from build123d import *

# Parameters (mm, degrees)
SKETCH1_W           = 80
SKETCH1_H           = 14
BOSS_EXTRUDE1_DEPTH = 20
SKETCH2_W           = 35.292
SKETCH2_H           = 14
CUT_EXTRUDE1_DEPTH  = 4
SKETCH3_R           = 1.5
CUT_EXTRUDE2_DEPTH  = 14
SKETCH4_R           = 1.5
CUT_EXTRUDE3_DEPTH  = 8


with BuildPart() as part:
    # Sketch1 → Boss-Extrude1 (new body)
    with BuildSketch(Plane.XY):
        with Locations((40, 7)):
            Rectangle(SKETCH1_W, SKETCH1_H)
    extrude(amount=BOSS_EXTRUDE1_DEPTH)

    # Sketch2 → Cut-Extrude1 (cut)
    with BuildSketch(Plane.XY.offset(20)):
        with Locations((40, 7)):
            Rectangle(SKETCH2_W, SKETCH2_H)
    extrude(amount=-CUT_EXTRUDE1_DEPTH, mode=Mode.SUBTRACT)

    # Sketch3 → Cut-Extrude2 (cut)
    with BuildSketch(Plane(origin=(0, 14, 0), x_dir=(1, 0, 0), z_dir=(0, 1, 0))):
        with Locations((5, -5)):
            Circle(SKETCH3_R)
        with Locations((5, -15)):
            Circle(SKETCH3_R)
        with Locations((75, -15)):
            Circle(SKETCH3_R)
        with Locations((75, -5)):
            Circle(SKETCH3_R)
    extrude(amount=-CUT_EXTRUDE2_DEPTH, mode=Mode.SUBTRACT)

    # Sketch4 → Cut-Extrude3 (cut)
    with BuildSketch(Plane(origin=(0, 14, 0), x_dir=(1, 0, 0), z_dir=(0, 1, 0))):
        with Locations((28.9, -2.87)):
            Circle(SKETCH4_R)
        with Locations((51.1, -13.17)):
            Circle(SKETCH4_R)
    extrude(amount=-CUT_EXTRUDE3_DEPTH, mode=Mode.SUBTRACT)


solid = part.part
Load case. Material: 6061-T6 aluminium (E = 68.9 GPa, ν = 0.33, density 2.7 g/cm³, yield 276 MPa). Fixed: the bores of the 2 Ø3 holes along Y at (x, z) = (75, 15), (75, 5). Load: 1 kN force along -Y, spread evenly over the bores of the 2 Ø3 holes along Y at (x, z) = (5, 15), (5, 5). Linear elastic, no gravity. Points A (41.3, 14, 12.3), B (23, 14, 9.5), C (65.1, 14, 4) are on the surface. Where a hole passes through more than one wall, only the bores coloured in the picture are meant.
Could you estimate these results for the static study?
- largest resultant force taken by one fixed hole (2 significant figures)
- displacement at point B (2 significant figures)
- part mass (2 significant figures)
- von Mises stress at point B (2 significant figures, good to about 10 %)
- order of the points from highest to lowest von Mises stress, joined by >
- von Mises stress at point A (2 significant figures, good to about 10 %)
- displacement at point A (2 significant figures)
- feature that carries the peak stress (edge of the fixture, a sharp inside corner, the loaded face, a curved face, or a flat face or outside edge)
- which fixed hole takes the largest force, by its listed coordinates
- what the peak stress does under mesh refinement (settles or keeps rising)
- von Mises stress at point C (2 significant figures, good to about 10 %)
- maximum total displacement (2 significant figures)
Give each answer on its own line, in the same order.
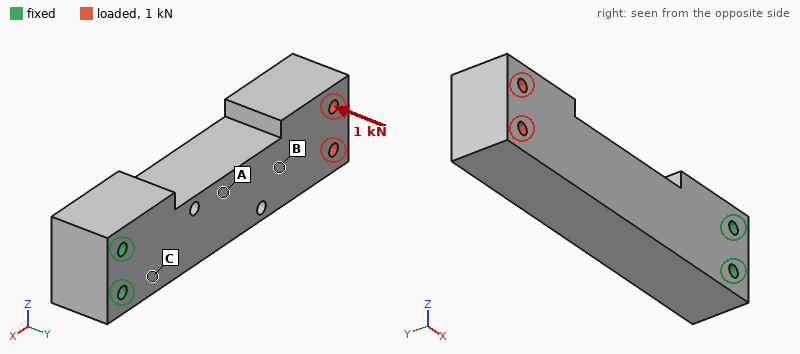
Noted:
570 N
0.28 mm
54 g
34 MPa
C > A > B
69 MPa
0.14 mm
edge of the fixture
(75, 15)
keeps rising
100 MPa
0.49 mm
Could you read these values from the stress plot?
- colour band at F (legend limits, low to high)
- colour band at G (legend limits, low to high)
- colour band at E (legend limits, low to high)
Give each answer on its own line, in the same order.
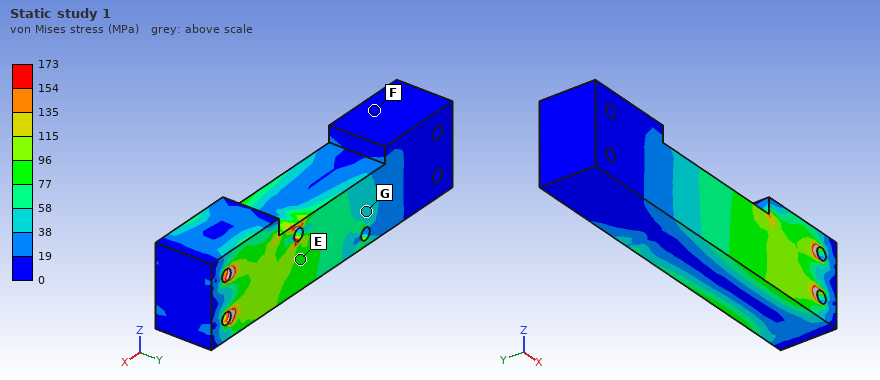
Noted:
0 to 19 MPa
38 to 58 MPa
77 to 96 MPa
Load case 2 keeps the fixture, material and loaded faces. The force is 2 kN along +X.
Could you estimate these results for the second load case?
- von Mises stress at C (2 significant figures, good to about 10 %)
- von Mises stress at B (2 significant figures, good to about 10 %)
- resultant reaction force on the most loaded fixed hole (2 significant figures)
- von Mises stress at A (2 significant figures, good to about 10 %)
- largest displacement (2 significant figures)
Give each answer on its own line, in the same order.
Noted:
7.0 MPa
9.0 MPa
1.0 kN
12 MPa
27 µm
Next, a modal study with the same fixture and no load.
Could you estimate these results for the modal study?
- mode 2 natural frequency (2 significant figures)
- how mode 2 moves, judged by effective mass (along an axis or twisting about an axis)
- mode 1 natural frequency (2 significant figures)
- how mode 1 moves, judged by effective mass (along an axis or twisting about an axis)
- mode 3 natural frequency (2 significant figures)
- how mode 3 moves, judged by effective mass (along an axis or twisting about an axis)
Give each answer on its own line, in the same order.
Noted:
2300 Hz
along Z
1900 Hz
along Y
8600 Hz
twisting about X
